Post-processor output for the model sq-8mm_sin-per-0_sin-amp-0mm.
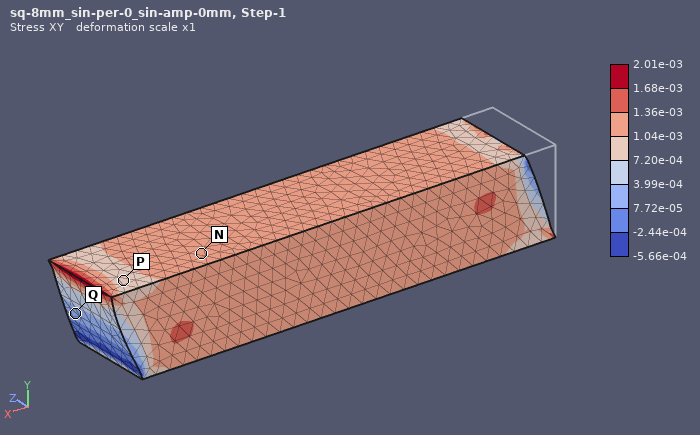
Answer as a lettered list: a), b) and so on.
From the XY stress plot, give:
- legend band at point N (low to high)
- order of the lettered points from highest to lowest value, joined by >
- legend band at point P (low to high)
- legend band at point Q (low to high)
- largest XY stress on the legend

a) 1.04e-03 to 1.36e-03
b) N > P > Q
c) 7.20e-04 to 1.04e-03
d) 7.72e-05 to 3.99e-04
e) 2.01e-03
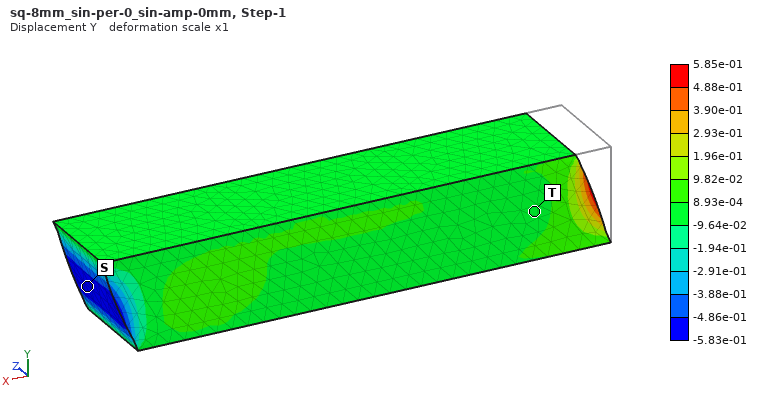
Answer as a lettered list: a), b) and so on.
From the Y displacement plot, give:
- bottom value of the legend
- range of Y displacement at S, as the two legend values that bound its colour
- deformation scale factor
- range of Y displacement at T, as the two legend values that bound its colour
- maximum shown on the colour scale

a) -5.83e-01
b) -5.83e-01 to -4.86e-01
c) 1
d) -9.64e-02 to 8.93e-04
e) 5.85e-01
